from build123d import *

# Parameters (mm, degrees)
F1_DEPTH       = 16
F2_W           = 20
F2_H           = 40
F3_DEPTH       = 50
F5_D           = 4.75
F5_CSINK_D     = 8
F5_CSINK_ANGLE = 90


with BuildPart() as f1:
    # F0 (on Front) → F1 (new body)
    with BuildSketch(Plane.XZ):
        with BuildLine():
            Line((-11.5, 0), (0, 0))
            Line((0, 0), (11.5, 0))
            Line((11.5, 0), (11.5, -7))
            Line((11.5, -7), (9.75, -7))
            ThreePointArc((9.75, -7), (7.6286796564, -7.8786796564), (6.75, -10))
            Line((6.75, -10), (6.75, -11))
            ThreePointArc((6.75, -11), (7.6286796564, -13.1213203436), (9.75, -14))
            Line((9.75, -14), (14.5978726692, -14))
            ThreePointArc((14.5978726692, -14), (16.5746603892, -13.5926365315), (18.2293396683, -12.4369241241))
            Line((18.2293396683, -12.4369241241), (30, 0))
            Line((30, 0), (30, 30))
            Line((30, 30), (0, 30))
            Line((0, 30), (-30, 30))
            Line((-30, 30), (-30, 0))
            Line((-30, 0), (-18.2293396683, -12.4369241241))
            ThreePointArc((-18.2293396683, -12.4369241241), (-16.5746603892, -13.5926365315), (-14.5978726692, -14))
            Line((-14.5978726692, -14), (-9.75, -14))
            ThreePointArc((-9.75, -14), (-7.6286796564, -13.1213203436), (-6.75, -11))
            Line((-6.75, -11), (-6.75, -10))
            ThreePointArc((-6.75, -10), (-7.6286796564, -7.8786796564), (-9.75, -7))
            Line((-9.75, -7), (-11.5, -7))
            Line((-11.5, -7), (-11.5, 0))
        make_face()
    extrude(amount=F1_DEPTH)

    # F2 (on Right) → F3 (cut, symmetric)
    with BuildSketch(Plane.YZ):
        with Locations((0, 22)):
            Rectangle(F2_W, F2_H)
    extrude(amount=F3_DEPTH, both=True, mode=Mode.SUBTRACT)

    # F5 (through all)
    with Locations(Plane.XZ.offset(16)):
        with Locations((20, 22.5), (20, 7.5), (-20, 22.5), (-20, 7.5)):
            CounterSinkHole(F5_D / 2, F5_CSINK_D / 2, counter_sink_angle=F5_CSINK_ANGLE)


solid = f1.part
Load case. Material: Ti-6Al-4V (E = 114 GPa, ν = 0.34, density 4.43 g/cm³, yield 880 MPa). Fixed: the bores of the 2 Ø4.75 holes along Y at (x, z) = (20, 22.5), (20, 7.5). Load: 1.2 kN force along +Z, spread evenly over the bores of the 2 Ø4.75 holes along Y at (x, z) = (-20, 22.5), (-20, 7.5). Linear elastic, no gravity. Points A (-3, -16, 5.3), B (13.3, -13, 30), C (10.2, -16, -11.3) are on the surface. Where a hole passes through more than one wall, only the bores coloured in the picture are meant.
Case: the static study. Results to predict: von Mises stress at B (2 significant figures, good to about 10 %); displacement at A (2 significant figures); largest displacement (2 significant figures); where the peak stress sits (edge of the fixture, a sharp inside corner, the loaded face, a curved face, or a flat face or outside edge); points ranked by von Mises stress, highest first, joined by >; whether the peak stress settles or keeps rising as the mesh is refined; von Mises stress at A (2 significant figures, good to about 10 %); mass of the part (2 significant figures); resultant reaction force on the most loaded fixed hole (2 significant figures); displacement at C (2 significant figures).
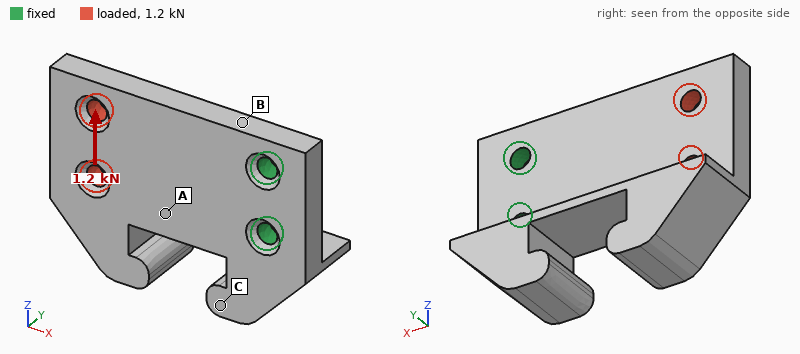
34 MPa
15 µm
46 µm
edge of the fixture
B > A > C
keeps rising
18 MPa
78 g
2.7 kN
9.3 µm
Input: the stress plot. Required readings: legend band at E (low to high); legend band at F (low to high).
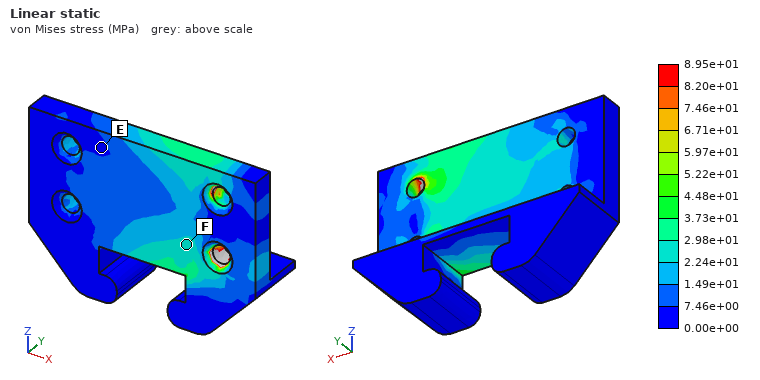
0.00e+00 to 7.46e+00 MPa
2.24e+01 to 2.98e+01 MPa
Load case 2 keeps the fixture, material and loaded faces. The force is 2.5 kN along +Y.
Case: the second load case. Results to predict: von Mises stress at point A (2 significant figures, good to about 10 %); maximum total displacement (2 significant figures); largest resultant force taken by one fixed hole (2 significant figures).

130 MPa
0.80 mm
1.3 kN
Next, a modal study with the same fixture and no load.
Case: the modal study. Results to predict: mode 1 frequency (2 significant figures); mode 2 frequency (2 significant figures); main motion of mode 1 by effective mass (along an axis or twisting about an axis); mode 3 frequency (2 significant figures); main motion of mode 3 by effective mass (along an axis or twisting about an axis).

1800 Hz
3400 Hz
along Y
5500 Hz
along Z
